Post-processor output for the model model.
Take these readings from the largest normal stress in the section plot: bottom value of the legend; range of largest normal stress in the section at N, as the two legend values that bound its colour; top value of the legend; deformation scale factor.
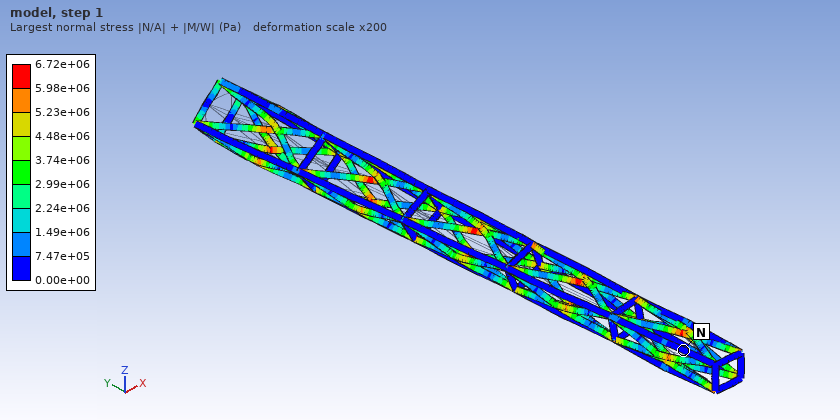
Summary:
0.00e+00 Pa
0.00e+00 to 7.47e+05 Pa
6.72e+06 Pa
200
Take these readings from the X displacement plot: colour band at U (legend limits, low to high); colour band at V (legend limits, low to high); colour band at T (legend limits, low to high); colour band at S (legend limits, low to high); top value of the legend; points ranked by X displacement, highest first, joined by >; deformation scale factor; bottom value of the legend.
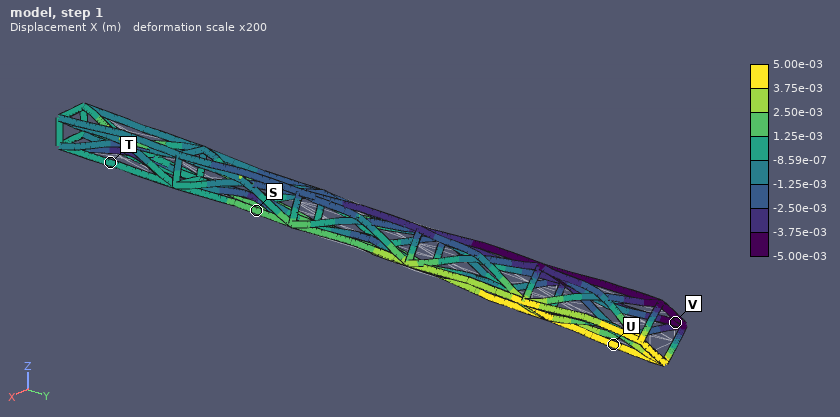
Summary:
3.75e-03 to 5.00e-03 m
-5.00e-03 to -3.75e-03 m
-8.59e-07 to 1.25e-03 m
1.25e-03 to 2.50e-03 m
5.00e-03 m
U > S > T > V
200
-5.00e-03 m
